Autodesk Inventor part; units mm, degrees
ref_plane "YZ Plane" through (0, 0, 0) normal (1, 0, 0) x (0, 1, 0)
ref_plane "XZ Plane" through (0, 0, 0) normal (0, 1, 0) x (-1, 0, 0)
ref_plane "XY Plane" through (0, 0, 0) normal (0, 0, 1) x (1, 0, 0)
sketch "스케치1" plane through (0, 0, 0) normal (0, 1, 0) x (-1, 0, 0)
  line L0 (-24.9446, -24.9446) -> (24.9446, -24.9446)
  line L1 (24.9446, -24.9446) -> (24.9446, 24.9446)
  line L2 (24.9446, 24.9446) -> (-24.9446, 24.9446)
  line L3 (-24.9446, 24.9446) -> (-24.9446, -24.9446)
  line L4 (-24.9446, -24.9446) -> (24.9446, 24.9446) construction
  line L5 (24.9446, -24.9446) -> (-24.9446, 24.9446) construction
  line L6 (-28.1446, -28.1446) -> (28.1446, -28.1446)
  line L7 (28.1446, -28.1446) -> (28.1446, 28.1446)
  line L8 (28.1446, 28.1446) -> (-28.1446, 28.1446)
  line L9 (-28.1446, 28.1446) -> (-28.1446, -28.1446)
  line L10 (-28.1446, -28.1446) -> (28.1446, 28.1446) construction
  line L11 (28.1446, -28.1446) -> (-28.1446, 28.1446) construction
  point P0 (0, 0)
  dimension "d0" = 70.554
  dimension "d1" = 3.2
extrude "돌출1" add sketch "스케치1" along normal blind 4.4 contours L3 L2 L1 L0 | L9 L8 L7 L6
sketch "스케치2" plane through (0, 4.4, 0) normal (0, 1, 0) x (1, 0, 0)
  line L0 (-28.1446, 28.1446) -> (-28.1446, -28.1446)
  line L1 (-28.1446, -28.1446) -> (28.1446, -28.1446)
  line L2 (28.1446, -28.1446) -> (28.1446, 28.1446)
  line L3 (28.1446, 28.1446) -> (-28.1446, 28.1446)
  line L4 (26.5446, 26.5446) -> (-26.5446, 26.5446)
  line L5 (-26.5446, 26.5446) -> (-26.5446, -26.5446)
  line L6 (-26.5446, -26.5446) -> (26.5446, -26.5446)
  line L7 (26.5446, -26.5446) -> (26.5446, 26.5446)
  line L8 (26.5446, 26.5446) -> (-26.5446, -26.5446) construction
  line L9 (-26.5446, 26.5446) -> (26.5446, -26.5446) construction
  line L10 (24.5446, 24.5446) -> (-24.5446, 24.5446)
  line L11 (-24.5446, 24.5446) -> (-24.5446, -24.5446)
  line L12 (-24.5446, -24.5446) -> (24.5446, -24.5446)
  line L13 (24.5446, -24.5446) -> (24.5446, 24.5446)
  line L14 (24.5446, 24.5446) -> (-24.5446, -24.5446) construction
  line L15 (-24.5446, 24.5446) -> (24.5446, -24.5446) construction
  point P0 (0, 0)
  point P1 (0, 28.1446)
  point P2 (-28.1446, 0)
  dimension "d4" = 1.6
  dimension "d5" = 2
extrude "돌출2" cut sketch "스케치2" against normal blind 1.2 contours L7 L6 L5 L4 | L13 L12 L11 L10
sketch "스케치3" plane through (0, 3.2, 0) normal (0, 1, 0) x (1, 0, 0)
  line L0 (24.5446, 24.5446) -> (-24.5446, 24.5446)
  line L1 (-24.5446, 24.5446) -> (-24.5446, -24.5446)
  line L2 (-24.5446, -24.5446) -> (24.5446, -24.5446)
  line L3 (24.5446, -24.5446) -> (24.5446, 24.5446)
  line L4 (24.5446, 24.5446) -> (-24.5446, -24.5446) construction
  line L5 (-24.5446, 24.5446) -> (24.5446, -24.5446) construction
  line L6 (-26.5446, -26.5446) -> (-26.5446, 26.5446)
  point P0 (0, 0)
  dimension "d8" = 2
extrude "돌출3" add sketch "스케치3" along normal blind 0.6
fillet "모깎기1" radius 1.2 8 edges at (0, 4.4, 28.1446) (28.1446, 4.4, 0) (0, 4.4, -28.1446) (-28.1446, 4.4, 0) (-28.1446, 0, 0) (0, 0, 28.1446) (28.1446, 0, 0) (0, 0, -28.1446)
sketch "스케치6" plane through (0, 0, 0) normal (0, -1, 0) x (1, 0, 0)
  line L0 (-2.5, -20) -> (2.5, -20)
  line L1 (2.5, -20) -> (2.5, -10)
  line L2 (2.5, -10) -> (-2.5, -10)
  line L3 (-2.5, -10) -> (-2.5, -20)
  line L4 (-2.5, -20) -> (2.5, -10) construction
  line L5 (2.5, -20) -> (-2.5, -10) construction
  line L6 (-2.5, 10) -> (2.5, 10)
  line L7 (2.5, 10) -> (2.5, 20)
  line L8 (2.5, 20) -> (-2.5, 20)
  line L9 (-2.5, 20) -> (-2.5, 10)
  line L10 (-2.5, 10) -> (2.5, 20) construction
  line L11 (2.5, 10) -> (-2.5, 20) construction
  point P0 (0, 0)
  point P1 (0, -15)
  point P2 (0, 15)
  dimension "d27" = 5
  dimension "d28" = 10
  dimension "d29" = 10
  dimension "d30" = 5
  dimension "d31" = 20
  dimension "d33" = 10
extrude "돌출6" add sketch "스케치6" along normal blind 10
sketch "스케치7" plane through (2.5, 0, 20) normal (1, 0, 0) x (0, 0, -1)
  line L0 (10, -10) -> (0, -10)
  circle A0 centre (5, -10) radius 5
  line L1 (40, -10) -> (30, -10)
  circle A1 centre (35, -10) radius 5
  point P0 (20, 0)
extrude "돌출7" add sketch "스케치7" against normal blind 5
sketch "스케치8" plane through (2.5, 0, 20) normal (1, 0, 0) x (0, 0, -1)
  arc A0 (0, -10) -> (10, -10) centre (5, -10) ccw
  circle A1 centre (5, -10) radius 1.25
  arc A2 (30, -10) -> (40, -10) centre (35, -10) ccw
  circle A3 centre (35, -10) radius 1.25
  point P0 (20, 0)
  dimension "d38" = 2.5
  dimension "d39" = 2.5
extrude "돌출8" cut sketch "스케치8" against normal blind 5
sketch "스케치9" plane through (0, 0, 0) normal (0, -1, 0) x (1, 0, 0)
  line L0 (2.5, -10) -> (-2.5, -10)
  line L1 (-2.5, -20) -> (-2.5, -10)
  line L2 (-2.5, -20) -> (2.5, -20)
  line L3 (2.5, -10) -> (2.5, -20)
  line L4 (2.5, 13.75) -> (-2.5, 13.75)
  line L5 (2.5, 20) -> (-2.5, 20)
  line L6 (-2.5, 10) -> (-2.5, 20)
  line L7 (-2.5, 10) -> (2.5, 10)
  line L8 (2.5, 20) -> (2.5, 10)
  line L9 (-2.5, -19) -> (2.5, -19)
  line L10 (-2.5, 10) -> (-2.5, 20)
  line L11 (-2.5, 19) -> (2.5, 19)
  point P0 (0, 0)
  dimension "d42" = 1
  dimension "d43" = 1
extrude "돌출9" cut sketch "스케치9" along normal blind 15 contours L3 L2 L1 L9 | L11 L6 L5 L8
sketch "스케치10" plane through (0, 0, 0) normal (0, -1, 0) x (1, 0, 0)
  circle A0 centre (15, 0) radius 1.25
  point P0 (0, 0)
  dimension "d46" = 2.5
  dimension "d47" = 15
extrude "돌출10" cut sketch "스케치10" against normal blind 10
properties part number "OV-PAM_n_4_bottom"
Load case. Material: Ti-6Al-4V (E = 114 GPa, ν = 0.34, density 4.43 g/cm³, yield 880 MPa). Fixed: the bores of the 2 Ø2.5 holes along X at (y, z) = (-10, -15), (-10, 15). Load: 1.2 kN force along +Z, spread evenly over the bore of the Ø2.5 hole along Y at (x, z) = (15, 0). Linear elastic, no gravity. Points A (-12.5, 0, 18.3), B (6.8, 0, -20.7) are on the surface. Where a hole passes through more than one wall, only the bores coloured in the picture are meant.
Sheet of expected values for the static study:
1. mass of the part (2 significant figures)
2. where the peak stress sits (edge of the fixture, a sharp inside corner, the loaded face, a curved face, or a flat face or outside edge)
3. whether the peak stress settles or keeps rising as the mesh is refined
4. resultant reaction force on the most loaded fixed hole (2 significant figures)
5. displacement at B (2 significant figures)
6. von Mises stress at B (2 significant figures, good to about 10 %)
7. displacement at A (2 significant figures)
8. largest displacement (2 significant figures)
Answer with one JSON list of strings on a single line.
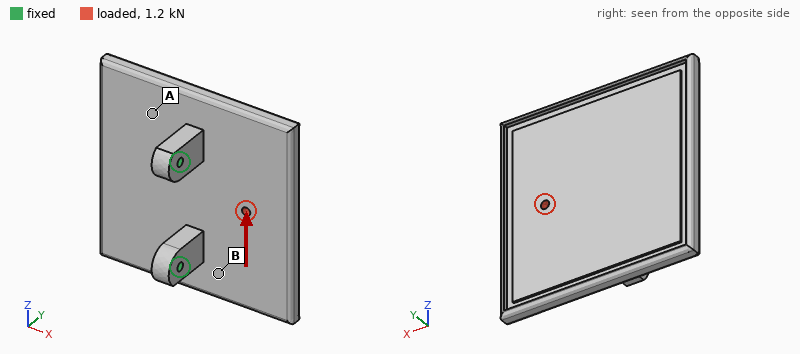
["58 g", "edge of the fixture", "keeps rising", "840 N", "29 µm", "24 MPa", "23 µm", "58 µm"]
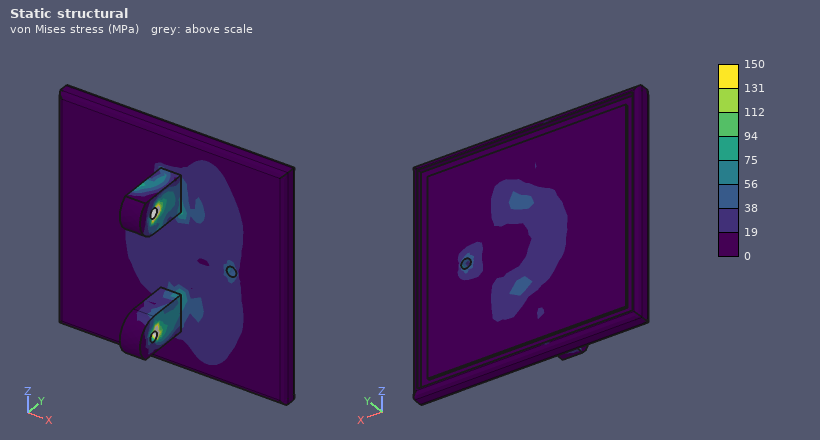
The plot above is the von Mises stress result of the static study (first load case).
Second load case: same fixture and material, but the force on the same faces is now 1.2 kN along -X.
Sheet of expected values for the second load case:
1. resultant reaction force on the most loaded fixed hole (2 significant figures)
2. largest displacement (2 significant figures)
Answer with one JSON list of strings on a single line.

["600 N", "0.12 mm"]
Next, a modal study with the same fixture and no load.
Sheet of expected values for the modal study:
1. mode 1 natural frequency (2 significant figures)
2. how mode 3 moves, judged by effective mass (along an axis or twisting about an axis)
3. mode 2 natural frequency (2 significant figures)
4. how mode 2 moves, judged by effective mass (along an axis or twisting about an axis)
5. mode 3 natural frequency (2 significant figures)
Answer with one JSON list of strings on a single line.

["1600 Hz", "along Y", "3400 Hz", "twisting about Y", "4200 Hz"]
